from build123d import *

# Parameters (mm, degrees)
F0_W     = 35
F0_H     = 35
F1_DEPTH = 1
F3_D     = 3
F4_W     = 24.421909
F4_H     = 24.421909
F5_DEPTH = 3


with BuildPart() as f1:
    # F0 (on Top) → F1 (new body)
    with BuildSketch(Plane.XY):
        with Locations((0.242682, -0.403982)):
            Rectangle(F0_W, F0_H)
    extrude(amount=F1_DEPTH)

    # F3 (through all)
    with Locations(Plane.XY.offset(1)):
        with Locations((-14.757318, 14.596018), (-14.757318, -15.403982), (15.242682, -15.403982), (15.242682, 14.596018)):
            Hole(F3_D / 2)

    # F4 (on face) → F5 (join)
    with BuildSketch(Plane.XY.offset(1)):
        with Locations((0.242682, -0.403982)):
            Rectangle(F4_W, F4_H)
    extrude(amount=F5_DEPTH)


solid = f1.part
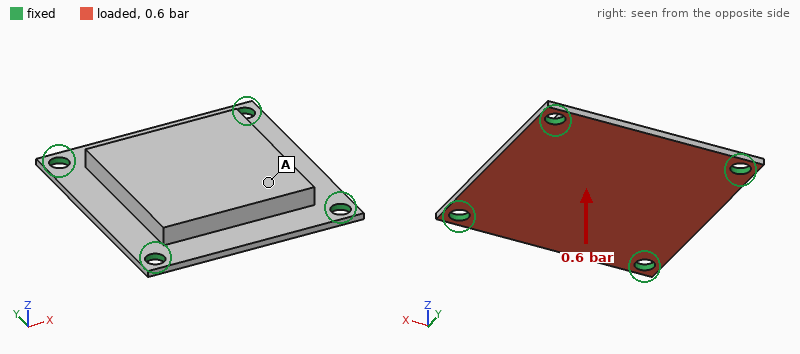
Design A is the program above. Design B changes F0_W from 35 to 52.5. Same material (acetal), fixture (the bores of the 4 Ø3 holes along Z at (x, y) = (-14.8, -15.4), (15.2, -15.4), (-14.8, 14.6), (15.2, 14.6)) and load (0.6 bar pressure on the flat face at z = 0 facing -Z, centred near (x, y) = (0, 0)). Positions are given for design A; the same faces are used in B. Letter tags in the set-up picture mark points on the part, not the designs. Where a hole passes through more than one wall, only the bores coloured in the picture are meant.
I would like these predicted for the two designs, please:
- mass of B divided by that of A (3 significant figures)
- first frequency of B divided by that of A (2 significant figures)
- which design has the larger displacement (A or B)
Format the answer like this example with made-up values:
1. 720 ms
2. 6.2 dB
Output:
1. 1.21
2. 0.74
3. B
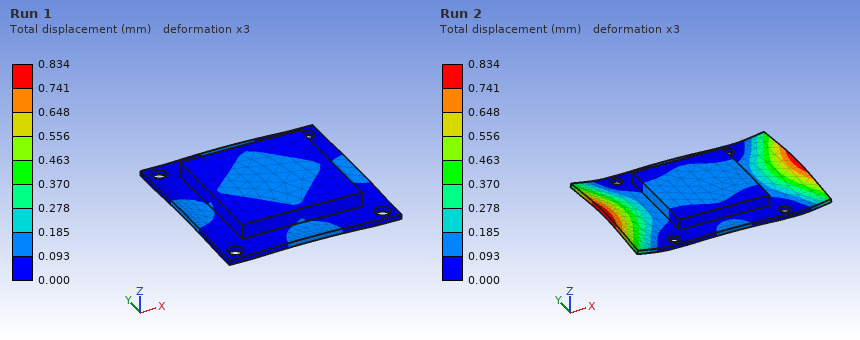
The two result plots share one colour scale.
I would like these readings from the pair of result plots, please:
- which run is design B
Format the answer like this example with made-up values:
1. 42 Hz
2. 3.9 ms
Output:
1. Run 2
